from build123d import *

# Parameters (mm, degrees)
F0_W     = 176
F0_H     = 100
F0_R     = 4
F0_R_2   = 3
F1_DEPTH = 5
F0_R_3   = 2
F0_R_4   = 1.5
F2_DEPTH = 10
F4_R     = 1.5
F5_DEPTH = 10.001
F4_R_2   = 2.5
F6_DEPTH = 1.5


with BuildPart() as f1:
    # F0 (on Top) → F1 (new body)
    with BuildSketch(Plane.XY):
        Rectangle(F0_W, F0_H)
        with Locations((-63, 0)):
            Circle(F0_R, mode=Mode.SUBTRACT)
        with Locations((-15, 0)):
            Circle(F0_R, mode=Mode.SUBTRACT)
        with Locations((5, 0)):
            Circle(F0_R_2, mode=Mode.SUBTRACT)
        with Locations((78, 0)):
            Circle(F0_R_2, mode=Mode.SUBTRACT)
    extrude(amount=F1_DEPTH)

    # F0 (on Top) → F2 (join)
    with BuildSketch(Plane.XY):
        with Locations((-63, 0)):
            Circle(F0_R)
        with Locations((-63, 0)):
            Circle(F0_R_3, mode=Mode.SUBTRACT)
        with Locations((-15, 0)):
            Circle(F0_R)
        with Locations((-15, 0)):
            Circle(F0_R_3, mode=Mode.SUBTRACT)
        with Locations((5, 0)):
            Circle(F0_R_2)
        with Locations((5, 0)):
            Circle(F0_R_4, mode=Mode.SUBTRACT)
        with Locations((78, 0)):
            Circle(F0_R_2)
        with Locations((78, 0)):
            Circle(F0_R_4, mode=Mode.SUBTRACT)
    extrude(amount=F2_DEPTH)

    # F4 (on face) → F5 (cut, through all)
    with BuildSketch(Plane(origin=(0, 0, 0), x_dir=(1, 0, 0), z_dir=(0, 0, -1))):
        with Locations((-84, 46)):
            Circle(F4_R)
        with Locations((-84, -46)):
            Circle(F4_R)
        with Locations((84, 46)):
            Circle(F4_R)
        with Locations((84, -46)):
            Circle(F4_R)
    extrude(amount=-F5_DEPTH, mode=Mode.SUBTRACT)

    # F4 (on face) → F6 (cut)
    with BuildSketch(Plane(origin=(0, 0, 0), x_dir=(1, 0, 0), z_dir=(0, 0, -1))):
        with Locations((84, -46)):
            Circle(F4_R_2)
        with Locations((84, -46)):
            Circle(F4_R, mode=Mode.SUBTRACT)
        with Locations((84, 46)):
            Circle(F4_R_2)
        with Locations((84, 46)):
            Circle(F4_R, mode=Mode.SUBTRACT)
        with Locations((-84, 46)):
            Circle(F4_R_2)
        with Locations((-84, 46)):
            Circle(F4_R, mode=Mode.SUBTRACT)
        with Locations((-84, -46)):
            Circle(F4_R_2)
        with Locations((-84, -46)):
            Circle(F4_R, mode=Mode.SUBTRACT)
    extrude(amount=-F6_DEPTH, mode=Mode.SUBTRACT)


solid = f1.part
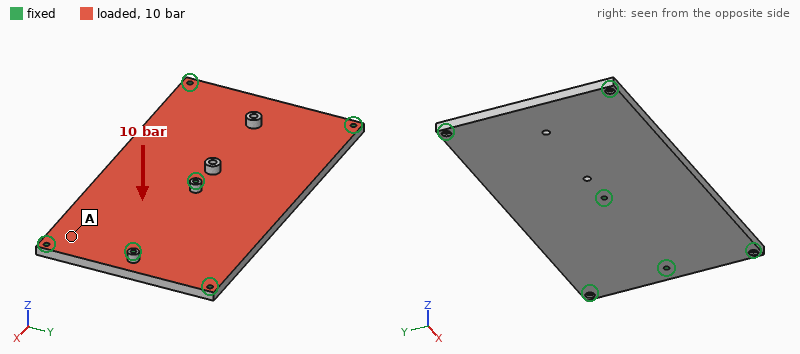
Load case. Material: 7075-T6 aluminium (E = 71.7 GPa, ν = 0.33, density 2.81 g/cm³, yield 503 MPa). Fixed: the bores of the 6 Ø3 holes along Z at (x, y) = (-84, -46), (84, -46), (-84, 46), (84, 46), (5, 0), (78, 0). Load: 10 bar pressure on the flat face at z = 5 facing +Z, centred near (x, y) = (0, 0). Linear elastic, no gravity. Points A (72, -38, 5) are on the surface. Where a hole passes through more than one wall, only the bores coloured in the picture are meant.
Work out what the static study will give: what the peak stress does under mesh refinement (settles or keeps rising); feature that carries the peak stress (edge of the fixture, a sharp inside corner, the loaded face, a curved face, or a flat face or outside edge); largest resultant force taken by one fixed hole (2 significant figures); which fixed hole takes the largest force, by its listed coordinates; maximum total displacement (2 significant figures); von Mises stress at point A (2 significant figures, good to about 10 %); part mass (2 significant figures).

keeps rising
edge of the fixture
8.7 kN
(5, 0)
0.85 mm
70 MPa
250 g
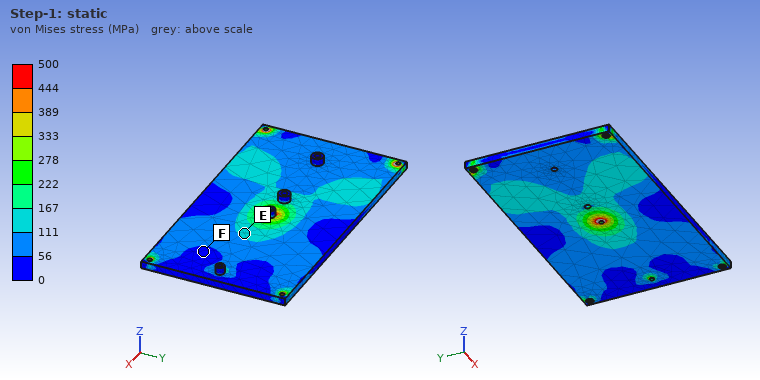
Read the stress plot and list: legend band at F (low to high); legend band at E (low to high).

0 to 56 MPa
111 to 167 MPa
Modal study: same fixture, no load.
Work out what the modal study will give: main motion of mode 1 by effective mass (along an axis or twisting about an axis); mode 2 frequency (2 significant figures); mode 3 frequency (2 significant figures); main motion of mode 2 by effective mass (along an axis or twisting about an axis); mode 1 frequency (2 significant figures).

twisting about X
1800 Hz
2200 Hz
along Z
1600 Hz
